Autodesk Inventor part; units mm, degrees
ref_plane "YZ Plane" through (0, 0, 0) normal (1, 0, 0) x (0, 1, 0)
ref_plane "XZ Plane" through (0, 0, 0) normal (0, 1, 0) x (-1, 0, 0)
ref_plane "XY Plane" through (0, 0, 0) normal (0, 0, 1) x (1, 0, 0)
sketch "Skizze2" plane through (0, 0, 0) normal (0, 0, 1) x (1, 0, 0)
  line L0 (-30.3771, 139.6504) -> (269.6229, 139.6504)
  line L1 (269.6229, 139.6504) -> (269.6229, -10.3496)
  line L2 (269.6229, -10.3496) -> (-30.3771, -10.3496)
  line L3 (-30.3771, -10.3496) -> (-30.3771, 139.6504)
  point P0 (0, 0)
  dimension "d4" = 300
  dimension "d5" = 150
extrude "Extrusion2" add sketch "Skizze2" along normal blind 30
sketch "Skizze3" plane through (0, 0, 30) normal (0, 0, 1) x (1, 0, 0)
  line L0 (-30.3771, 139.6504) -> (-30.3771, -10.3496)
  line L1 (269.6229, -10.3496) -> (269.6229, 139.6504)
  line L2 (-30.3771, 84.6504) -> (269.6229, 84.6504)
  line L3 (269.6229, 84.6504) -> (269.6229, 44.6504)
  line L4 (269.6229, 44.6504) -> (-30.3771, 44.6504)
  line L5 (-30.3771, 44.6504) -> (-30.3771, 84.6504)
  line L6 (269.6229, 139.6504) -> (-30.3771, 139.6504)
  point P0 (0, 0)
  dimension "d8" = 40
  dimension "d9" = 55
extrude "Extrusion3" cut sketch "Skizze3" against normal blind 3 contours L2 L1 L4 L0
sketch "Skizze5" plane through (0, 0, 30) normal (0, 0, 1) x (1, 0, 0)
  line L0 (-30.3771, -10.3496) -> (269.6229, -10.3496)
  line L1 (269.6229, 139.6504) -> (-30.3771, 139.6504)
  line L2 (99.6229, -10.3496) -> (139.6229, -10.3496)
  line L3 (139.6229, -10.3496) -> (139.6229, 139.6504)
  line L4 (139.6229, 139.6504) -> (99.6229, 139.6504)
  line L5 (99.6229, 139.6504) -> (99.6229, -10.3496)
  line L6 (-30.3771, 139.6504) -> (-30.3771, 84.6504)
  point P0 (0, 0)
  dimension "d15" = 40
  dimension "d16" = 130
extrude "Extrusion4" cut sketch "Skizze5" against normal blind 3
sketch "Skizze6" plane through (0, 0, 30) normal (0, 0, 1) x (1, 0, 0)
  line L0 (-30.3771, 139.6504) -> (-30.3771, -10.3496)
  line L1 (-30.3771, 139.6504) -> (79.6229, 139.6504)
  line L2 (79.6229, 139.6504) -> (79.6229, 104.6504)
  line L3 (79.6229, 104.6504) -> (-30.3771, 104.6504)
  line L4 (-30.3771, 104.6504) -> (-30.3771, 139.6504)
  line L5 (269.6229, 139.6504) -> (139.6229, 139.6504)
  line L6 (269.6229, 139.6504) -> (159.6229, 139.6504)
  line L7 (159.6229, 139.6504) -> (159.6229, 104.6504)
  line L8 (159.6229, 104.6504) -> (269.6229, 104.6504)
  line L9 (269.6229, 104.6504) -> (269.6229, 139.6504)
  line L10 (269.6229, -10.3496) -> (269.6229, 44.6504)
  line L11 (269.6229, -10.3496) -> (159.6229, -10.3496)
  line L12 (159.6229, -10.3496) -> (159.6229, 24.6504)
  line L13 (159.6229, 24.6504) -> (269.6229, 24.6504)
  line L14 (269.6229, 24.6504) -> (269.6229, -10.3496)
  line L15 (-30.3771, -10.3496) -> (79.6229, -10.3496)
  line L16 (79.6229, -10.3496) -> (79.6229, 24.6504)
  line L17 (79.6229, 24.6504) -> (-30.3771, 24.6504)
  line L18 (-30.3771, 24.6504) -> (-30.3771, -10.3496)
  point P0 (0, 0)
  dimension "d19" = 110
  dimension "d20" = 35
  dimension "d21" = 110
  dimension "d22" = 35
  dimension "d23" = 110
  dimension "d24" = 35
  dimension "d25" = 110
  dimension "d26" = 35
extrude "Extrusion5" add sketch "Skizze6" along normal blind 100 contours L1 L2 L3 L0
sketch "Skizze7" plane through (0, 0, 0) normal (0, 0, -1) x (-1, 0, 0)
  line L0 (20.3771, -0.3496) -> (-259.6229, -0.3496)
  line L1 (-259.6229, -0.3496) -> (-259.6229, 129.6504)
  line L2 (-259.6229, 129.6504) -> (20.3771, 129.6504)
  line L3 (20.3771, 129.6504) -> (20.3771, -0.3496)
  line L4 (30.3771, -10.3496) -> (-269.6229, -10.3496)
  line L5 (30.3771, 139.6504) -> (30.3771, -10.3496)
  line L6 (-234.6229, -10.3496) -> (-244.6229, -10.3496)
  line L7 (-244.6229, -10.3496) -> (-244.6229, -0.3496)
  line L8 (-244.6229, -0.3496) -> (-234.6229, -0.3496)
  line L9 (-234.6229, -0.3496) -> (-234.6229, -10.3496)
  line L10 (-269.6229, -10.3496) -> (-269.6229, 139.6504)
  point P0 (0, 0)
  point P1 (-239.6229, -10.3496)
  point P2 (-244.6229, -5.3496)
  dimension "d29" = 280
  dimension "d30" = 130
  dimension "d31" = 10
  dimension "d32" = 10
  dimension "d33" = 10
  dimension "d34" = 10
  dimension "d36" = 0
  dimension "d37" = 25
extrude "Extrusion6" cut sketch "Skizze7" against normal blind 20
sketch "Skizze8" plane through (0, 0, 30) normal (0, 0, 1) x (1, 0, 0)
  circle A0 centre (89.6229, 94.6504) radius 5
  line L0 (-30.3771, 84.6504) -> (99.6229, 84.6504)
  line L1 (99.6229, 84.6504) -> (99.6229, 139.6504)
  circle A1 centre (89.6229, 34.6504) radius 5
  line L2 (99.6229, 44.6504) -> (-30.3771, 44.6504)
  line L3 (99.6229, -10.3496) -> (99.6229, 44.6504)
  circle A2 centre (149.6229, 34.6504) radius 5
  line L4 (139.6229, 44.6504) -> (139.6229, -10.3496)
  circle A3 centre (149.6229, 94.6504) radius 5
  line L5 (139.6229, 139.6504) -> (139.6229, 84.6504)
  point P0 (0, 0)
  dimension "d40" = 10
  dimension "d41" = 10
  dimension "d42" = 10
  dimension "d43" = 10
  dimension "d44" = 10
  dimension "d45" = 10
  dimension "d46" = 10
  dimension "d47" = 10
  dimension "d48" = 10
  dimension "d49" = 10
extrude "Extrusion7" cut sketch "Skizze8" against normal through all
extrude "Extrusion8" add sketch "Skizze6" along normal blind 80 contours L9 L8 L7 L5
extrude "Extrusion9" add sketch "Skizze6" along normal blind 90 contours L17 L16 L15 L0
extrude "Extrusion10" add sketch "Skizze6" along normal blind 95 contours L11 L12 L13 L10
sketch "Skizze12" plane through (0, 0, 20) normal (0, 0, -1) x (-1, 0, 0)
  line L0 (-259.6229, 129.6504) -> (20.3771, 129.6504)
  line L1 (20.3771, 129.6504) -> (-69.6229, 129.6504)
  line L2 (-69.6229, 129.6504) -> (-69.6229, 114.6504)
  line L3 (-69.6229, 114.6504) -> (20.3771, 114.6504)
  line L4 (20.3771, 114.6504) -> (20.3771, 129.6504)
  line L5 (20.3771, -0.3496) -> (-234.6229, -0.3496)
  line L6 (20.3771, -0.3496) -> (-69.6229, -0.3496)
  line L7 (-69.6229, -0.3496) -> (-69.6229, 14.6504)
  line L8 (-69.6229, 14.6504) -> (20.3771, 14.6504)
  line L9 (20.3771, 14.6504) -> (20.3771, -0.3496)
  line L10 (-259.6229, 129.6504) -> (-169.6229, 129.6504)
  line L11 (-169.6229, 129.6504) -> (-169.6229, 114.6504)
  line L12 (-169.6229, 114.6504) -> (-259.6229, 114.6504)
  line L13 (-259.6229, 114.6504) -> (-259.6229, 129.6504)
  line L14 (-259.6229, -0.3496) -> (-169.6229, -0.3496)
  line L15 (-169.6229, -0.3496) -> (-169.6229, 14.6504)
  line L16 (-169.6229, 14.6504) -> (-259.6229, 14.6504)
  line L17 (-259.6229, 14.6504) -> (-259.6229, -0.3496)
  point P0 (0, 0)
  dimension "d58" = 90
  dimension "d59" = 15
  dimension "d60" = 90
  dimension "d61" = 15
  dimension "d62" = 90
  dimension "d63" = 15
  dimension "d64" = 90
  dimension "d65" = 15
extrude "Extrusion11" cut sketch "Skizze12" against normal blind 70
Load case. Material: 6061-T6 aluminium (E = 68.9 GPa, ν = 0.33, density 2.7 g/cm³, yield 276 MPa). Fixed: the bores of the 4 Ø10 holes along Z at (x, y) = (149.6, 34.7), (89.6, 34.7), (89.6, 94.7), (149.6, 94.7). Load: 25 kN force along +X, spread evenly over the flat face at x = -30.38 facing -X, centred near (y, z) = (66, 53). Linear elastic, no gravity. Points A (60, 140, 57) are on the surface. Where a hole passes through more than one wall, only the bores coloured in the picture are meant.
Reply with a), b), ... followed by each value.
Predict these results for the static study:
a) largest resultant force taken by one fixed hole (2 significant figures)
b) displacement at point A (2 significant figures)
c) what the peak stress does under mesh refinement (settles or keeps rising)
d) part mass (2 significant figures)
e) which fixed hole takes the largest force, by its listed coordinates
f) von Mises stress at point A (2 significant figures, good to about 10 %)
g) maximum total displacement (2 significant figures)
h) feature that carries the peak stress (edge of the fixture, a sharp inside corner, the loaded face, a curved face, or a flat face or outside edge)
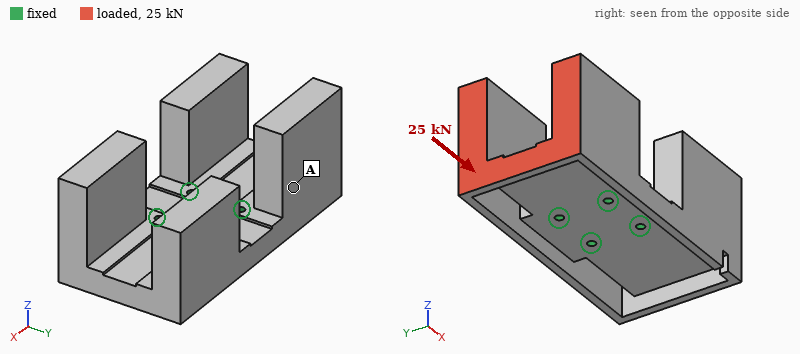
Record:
a) 13 kN
b) 0.46 mm
c) keeps rising
d) 4.3 kg
e) (89.6, 94.7)
f) 18 MPa
g) 1.5 mm
h) edge of the fixture
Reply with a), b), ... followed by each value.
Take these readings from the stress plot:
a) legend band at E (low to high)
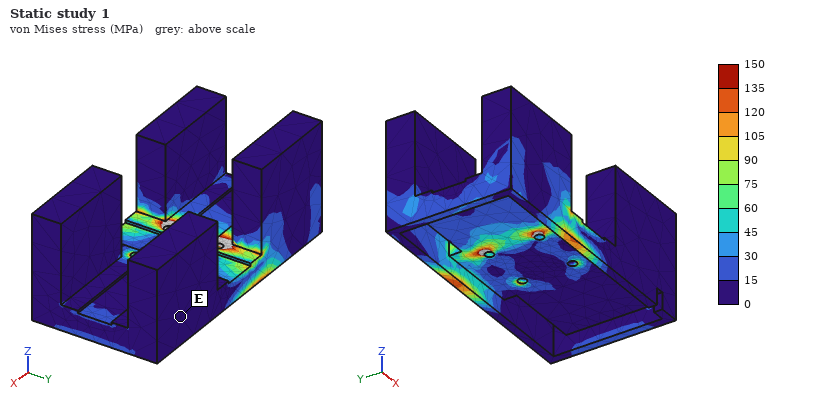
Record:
a) 0 to 15 MPa
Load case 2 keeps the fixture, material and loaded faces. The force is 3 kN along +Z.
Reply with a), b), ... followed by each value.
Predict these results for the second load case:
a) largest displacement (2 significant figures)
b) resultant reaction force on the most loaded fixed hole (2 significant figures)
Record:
a) 0.73 mm
b) 3.6 kN
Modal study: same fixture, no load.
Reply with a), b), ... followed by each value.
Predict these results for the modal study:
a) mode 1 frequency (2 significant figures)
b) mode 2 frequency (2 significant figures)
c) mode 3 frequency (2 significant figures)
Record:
a) 310 Hz
b) 330 Hz
c) 360 Hz
